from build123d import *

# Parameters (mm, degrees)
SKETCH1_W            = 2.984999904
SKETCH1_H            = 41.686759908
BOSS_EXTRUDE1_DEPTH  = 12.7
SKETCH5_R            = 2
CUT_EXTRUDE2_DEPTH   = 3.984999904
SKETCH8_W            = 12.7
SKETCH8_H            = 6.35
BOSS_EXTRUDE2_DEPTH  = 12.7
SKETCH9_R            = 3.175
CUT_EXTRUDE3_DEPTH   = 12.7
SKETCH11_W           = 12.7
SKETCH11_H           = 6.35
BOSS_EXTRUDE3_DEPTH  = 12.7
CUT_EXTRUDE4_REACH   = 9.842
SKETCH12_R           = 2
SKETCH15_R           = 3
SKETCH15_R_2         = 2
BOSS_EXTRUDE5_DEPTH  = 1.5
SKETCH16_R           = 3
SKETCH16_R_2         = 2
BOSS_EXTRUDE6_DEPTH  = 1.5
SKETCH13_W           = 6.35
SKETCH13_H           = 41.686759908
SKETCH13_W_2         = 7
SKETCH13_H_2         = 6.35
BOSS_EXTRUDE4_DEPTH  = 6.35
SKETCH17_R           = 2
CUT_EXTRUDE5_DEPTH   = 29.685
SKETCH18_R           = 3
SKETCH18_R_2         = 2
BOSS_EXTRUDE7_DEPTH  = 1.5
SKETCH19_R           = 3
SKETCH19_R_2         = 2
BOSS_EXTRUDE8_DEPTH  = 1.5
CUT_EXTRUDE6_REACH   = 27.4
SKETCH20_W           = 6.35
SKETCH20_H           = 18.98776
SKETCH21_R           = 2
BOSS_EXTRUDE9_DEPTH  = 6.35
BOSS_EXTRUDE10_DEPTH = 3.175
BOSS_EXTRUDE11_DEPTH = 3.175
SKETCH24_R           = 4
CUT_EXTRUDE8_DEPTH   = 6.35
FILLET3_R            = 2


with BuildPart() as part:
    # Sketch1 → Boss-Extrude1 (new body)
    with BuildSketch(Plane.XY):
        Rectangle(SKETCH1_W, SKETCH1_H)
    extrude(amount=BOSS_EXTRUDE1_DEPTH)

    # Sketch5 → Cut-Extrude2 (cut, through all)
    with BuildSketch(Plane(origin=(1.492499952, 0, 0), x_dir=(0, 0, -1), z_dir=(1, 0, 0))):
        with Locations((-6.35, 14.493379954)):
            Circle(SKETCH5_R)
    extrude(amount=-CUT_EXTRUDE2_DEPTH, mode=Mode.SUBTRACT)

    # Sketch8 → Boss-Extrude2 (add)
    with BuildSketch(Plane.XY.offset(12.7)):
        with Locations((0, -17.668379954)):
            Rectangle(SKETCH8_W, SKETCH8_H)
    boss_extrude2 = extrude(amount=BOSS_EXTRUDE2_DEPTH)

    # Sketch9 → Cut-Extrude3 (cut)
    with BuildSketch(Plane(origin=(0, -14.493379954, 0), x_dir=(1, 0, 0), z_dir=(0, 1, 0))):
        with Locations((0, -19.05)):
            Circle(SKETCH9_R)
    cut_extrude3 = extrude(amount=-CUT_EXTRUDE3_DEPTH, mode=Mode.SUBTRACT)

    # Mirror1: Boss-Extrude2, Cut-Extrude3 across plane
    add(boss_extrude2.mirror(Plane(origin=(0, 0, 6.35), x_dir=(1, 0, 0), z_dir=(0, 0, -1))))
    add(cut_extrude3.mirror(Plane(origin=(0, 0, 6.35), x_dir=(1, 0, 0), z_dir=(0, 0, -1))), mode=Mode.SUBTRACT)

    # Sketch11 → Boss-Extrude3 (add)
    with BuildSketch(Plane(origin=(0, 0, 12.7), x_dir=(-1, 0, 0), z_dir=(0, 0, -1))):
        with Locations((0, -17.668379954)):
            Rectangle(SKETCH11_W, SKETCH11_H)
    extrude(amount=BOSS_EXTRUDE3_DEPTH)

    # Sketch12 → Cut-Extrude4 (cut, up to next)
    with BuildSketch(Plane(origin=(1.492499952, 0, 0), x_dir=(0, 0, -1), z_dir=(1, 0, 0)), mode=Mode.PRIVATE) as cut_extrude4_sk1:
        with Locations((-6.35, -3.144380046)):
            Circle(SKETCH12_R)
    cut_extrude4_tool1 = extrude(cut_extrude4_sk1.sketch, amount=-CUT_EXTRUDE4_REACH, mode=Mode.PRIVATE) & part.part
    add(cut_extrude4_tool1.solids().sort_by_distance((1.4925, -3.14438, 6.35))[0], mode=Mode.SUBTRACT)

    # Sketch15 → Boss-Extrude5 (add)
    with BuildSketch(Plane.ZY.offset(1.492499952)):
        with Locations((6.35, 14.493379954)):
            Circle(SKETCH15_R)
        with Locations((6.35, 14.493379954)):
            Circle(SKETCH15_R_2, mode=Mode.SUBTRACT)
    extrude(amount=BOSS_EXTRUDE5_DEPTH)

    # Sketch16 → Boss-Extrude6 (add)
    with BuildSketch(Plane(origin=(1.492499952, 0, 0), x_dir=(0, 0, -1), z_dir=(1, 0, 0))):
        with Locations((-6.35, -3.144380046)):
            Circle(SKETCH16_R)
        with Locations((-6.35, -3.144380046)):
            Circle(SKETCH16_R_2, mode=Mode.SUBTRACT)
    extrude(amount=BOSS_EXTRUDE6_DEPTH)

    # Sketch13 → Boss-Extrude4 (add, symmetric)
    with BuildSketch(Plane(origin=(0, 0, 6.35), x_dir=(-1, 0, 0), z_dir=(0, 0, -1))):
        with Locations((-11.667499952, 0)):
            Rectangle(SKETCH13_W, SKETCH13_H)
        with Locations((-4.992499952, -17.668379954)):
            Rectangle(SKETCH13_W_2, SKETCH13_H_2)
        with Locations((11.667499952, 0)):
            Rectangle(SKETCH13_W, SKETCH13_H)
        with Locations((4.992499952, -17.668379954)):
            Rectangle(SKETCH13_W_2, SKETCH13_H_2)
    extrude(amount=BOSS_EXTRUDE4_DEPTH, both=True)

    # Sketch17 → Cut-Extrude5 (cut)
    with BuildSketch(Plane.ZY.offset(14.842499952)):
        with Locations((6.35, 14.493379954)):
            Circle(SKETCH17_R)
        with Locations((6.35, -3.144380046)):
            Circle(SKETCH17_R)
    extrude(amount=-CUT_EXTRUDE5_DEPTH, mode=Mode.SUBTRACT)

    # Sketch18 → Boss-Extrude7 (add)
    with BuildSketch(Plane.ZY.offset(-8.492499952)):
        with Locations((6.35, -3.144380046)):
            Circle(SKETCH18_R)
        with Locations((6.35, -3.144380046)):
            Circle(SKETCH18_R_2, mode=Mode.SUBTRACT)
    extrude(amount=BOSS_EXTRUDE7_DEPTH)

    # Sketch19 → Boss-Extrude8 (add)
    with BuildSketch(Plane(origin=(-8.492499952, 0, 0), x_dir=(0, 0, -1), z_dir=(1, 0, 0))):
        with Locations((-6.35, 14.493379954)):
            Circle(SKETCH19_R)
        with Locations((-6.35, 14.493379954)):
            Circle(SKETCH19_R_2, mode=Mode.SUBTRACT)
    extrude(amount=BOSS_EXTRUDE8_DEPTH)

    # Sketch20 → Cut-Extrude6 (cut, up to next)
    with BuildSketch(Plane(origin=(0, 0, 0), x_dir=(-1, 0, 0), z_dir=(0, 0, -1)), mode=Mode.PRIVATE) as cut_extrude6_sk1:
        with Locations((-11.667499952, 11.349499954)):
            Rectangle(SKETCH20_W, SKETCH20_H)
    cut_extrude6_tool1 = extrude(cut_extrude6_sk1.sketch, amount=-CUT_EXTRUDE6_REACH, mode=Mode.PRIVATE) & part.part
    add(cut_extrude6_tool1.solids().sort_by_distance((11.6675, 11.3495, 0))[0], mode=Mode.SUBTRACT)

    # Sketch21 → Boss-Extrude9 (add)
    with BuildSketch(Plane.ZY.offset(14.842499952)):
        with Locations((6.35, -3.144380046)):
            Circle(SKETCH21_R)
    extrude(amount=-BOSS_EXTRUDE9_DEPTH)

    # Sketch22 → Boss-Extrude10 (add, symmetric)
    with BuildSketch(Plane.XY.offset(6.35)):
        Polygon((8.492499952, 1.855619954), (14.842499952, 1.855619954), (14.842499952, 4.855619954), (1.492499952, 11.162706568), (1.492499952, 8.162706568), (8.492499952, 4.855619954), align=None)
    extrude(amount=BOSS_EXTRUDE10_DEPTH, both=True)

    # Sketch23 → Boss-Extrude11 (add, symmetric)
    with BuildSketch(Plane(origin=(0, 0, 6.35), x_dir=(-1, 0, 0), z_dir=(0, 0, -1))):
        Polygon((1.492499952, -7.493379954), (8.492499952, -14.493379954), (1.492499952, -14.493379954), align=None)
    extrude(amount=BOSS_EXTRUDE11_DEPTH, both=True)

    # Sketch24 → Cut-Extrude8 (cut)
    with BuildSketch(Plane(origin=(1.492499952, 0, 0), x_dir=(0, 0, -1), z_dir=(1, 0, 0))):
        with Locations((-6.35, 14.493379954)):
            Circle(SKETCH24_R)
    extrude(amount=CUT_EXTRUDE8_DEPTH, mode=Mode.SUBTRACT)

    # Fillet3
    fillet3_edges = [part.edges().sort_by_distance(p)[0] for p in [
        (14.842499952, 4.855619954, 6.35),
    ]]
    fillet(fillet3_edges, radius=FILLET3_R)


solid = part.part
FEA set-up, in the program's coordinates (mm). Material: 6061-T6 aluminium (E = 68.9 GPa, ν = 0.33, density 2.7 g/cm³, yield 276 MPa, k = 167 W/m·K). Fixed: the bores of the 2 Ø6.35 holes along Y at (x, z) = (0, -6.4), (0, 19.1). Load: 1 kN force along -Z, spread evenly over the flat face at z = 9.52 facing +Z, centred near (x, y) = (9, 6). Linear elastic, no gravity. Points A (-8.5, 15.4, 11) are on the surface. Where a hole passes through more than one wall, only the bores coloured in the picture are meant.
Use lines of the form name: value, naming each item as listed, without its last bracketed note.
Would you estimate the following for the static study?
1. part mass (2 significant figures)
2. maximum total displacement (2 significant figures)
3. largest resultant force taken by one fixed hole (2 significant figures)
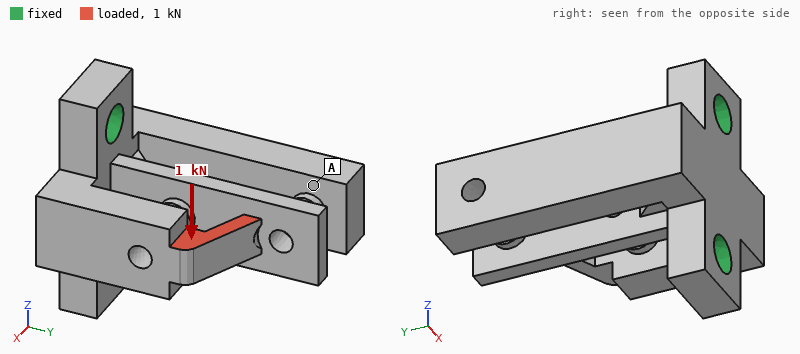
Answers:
part mass: 27 g
maximum total displacement: 0.15 mm
largest resultant force taken by one fixed hole: 1.5 kN
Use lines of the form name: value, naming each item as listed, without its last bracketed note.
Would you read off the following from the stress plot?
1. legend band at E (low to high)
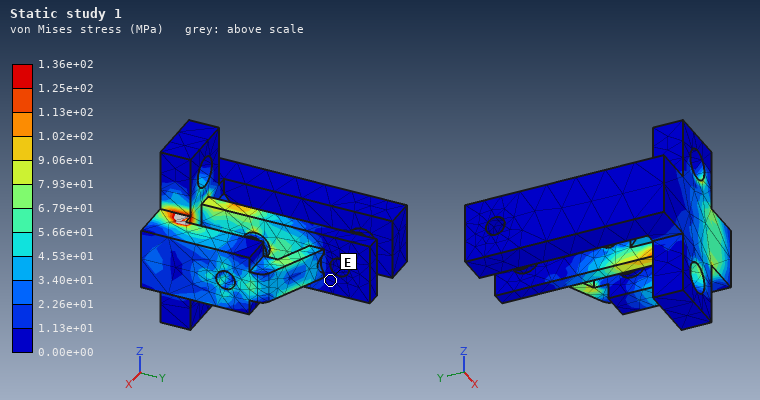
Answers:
legend band at E: 0.00e+00 to 1.13e+01 MPa
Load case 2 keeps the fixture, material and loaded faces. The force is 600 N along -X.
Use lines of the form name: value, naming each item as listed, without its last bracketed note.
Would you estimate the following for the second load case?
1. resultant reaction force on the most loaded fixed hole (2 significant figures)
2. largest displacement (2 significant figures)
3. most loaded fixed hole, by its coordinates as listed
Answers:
resultant reaction force on the most loaded fixed hole: 390 N
largest displacement: 0.25 mm
most loaded fixed hole, by its coordinates as listed: (0, 19.1)
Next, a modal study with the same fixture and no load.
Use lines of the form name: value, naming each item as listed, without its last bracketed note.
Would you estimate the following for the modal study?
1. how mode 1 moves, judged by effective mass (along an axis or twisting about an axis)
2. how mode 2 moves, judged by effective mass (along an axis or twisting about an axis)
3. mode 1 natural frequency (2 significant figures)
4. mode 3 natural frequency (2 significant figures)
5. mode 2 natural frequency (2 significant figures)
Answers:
how mode 1 moves, judged by effective mass: along X
how mode 2 moves, judged by effective mass: along Z
mode 1 natural frequency: 2600 Hz
mode 3 natural frequency: 4400 Hz
mode 2 natural frequency: 4200 Hz
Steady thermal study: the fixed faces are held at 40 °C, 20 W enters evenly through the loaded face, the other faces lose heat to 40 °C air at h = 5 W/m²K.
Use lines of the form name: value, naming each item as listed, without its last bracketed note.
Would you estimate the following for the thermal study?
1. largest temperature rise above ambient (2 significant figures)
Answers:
largest temperature rise above ambient: 44 K
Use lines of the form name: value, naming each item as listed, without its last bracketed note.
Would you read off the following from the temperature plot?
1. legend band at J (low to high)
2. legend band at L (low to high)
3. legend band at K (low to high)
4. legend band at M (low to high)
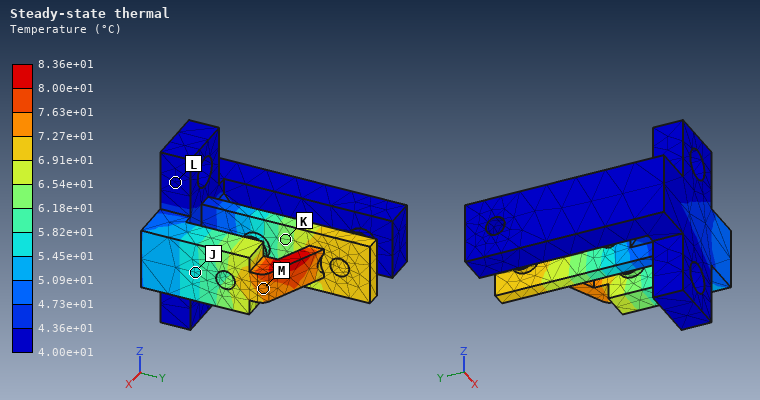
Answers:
legend band at J: 5.45e+01 to 5.82e+01 °C
legend band at L: 4.00e+01 to 4.36e+01 °C
legend band at K: 6.18e+01 to 6.54e+01 °C
legend band at M: 7.27e+01 to 7.63e+01 °C
